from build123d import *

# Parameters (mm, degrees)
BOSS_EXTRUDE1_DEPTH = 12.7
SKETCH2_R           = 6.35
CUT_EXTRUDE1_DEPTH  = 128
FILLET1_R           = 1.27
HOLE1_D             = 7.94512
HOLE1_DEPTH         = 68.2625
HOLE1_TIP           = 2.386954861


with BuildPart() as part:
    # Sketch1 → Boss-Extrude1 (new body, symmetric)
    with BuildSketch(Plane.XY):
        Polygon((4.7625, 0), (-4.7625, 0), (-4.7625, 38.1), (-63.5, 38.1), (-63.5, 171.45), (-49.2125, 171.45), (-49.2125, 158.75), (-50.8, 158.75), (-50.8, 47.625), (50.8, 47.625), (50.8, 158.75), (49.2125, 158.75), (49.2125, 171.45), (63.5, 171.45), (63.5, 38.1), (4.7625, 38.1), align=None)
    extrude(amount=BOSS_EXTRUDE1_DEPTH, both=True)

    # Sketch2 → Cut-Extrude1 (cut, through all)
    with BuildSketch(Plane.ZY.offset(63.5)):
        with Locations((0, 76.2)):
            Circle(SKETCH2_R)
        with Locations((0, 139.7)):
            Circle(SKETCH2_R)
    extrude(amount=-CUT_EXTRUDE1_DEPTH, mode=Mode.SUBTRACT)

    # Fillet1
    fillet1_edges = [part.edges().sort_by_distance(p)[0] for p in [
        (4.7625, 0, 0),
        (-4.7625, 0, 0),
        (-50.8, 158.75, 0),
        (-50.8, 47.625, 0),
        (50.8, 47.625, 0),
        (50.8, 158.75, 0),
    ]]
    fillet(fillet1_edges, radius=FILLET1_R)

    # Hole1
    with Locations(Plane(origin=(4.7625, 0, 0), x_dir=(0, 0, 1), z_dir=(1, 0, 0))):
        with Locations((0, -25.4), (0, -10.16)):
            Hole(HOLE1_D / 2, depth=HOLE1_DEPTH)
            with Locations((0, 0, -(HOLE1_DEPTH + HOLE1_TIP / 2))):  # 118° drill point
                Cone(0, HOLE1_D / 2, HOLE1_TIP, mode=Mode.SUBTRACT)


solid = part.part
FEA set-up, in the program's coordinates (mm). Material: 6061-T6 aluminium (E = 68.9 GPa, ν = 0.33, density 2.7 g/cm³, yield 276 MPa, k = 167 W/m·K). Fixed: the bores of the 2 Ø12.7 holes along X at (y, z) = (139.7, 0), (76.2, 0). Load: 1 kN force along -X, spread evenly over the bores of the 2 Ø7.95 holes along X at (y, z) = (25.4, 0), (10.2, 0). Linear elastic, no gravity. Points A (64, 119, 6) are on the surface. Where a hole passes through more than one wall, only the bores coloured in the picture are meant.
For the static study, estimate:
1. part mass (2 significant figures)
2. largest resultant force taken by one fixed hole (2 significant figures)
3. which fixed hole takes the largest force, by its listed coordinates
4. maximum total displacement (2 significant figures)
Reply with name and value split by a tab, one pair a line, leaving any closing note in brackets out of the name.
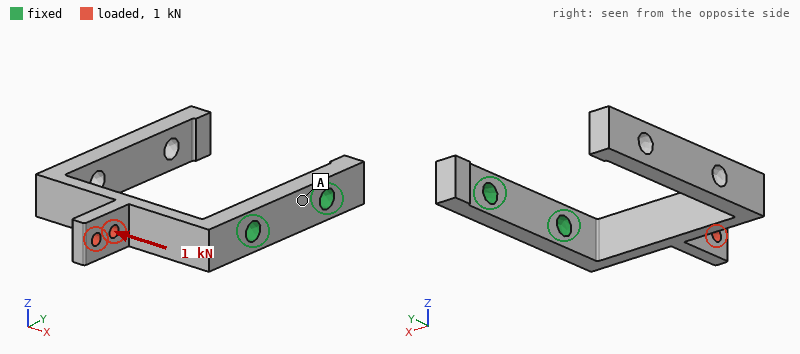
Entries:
part mass	310 g
largest resultant force taken by one fixed hole	1.0 kN
which fixed hole takes the largest force, by its listed coordinates	(76.2, 0)
maximum total displacement	2.2 mm
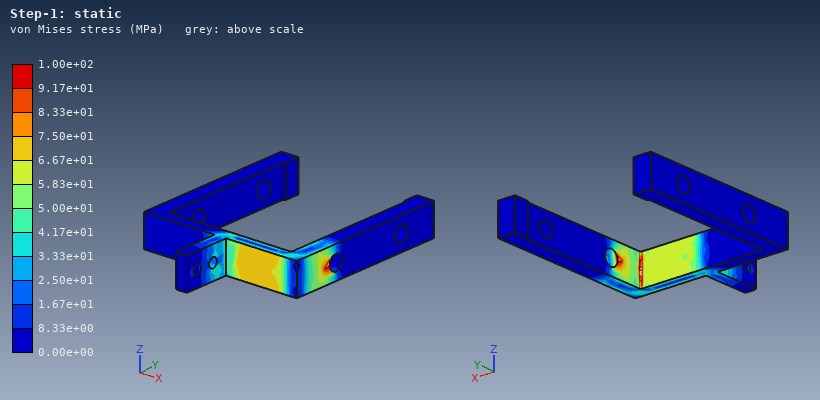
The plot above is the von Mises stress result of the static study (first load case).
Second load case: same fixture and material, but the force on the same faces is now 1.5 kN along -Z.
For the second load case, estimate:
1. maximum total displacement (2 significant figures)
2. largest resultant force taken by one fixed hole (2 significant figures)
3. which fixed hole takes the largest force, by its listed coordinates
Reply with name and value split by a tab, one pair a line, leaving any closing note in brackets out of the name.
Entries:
maximum total displacement	1.1 mm
largest resultant force taken by one fixed hole	1.7 kN
which fixed hole takes the largest force, by its listed coordinates	(76.2, 0)
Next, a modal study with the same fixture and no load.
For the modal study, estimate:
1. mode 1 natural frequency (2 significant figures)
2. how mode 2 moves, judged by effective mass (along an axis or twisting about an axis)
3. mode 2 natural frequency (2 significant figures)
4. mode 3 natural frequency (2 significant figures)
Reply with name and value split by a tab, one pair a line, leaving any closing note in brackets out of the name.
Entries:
mode 1 natural frequency	150 Hz
how mode 2 moves, judged by effective mass	along Z
mode 2 natural frequency	210 Hz
mode 3 natural frequency	440 Hz
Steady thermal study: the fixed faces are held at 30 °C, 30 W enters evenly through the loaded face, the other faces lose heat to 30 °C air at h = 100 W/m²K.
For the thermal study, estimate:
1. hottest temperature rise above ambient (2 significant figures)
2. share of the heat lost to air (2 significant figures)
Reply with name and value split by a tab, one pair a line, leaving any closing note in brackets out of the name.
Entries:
hottest temperature rise above ambient	33 K
share of the heat lost to air	72 %
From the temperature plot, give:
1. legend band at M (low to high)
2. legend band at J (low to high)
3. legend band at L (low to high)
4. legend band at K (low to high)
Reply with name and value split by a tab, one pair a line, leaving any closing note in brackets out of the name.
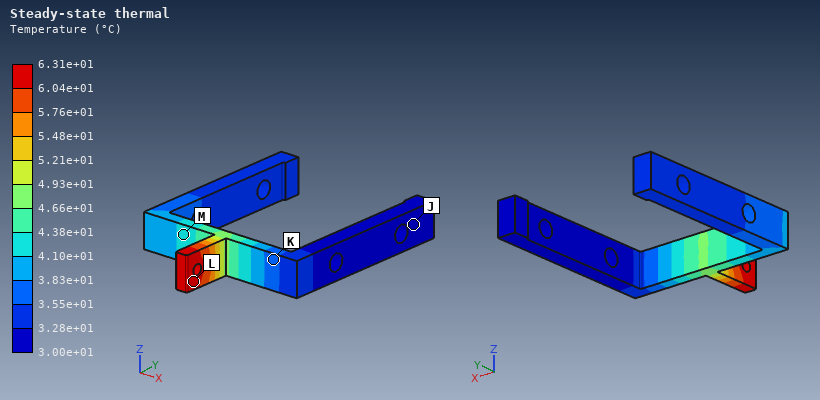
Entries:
legend band at M	4.10e+01 to 4.38e+01 °C
legend band at J	3.00e+01 to 3.28e+01 °C
legend band at L	6.04e+01 to 6.31e+01 °C
legend band at K	3.55e+01 to 3.83e+01 °C
